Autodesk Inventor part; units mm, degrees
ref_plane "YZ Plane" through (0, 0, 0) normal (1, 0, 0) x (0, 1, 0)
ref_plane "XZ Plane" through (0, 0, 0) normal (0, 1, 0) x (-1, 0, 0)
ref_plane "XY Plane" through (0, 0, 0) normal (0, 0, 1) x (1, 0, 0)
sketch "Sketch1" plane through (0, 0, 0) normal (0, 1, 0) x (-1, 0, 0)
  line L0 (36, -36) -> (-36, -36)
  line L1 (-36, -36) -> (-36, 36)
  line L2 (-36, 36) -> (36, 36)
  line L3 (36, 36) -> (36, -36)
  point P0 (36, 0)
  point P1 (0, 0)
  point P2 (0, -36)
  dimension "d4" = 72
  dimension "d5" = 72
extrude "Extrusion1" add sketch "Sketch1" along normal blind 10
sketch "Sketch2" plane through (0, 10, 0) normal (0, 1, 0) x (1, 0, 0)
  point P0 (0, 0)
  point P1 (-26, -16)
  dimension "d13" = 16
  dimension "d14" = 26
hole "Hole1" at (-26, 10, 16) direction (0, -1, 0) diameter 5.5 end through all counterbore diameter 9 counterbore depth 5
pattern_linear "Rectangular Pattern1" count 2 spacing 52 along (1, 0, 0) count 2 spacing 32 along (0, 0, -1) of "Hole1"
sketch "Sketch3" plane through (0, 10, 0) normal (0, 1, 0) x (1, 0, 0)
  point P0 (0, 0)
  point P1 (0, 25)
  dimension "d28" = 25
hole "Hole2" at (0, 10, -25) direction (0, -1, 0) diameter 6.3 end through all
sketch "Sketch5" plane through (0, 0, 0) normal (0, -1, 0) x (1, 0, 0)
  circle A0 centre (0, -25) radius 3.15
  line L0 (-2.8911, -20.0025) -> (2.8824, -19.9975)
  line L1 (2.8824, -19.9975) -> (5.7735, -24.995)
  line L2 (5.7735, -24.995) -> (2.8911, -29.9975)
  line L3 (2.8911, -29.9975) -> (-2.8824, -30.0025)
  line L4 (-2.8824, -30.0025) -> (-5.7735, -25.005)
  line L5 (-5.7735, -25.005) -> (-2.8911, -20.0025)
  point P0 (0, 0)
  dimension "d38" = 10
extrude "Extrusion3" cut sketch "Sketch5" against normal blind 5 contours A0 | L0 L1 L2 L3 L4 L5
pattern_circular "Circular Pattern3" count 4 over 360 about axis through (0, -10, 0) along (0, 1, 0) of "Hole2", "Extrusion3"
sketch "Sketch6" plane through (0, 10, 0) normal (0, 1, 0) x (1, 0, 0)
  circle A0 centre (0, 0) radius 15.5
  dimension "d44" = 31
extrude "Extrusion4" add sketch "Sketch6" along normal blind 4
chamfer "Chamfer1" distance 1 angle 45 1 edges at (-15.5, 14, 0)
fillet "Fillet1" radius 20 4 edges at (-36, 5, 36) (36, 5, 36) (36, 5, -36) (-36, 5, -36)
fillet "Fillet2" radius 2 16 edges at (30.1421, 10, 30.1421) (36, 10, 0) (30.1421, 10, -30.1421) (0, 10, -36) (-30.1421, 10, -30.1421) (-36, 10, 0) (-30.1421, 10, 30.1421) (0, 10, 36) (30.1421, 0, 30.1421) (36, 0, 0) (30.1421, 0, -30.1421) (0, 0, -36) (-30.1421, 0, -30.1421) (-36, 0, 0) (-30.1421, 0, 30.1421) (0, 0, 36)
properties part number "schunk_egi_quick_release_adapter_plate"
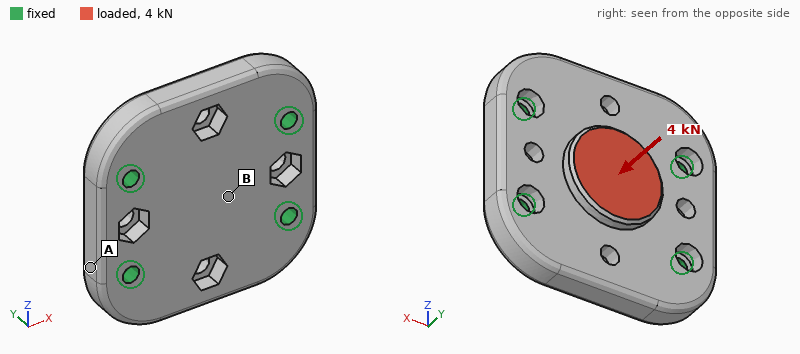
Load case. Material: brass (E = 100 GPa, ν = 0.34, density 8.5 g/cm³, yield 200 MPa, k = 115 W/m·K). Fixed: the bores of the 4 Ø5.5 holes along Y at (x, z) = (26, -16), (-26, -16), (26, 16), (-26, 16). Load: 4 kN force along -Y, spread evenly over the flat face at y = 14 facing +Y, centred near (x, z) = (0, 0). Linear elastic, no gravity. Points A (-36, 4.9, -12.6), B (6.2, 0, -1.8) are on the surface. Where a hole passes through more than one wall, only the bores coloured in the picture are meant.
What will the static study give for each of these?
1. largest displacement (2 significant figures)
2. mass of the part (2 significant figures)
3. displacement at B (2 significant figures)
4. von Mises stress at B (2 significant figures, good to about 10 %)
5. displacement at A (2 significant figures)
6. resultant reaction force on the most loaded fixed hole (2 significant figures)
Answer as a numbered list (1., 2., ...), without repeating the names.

1. 9.6 µm
2. 400 g
3. 8.9 µm
4. 14 MPa
5. 1.5 µm
6. 1.3 kN
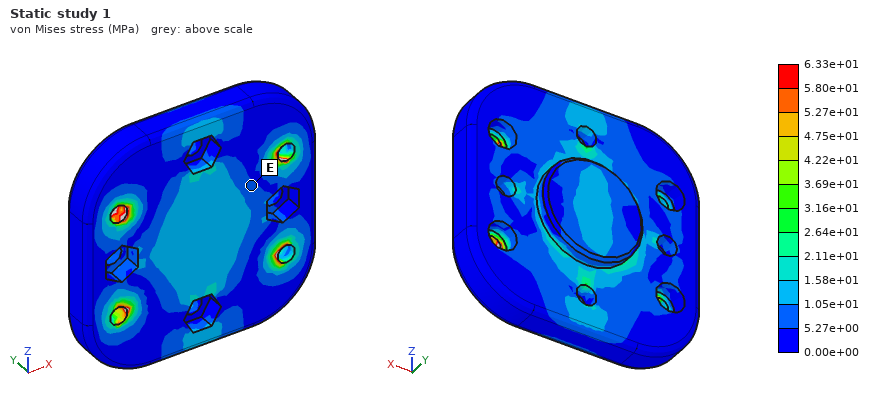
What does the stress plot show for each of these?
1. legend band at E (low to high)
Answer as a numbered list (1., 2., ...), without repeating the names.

1. 5.27e+00 to 1.05e+01 MPa
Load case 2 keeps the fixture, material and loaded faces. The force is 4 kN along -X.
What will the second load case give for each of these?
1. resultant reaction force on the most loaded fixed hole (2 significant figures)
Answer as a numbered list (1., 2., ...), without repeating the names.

1. 1.2 kN
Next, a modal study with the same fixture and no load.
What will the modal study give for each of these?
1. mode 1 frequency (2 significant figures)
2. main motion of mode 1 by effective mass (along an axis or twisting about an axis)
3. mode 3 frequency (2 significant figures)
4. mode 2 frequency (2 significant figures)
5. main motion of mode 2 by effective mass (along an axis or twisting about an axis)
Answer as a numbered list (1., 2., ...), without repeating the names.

1. 6600 Hz
2. twisting about X
3. 11 kHz
4. 6900 Hz
5. along Y
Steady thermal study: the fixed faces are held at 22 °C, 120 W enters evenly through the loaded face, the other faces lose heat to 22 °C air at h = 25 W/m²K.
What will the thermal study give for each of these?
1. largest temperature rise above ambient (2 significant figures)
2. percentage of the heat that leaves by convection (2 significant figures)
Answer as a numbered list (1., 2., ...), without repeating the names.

1. 37 K
2. 3.2 %
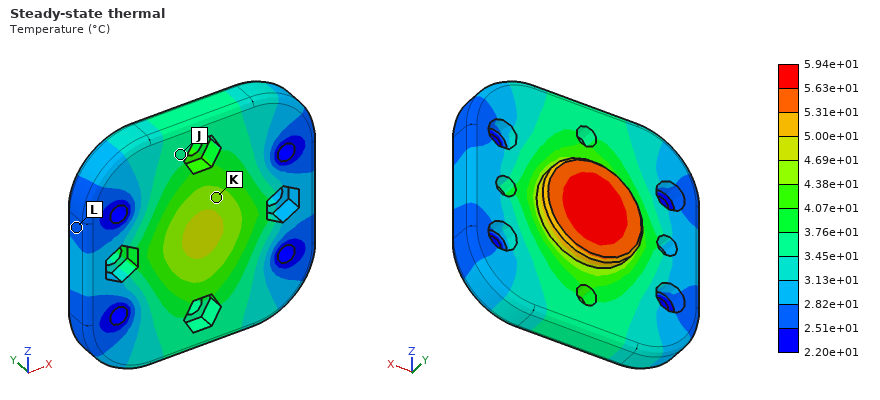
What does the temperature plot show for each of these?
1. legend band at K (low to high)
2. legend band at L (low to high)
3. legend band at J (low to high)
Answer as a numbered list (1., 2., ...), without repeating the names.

1. 4.38e+01 to 4.69e+01 °C
2. 2.51e+01 to 2.82e+01 °C
3. 3.45e+01 to 3.76e+01 °C
